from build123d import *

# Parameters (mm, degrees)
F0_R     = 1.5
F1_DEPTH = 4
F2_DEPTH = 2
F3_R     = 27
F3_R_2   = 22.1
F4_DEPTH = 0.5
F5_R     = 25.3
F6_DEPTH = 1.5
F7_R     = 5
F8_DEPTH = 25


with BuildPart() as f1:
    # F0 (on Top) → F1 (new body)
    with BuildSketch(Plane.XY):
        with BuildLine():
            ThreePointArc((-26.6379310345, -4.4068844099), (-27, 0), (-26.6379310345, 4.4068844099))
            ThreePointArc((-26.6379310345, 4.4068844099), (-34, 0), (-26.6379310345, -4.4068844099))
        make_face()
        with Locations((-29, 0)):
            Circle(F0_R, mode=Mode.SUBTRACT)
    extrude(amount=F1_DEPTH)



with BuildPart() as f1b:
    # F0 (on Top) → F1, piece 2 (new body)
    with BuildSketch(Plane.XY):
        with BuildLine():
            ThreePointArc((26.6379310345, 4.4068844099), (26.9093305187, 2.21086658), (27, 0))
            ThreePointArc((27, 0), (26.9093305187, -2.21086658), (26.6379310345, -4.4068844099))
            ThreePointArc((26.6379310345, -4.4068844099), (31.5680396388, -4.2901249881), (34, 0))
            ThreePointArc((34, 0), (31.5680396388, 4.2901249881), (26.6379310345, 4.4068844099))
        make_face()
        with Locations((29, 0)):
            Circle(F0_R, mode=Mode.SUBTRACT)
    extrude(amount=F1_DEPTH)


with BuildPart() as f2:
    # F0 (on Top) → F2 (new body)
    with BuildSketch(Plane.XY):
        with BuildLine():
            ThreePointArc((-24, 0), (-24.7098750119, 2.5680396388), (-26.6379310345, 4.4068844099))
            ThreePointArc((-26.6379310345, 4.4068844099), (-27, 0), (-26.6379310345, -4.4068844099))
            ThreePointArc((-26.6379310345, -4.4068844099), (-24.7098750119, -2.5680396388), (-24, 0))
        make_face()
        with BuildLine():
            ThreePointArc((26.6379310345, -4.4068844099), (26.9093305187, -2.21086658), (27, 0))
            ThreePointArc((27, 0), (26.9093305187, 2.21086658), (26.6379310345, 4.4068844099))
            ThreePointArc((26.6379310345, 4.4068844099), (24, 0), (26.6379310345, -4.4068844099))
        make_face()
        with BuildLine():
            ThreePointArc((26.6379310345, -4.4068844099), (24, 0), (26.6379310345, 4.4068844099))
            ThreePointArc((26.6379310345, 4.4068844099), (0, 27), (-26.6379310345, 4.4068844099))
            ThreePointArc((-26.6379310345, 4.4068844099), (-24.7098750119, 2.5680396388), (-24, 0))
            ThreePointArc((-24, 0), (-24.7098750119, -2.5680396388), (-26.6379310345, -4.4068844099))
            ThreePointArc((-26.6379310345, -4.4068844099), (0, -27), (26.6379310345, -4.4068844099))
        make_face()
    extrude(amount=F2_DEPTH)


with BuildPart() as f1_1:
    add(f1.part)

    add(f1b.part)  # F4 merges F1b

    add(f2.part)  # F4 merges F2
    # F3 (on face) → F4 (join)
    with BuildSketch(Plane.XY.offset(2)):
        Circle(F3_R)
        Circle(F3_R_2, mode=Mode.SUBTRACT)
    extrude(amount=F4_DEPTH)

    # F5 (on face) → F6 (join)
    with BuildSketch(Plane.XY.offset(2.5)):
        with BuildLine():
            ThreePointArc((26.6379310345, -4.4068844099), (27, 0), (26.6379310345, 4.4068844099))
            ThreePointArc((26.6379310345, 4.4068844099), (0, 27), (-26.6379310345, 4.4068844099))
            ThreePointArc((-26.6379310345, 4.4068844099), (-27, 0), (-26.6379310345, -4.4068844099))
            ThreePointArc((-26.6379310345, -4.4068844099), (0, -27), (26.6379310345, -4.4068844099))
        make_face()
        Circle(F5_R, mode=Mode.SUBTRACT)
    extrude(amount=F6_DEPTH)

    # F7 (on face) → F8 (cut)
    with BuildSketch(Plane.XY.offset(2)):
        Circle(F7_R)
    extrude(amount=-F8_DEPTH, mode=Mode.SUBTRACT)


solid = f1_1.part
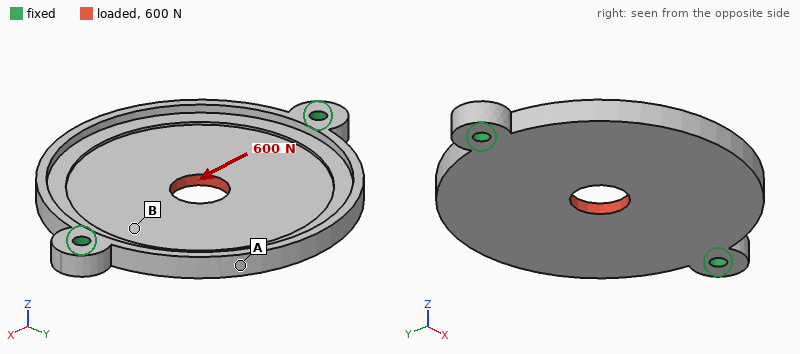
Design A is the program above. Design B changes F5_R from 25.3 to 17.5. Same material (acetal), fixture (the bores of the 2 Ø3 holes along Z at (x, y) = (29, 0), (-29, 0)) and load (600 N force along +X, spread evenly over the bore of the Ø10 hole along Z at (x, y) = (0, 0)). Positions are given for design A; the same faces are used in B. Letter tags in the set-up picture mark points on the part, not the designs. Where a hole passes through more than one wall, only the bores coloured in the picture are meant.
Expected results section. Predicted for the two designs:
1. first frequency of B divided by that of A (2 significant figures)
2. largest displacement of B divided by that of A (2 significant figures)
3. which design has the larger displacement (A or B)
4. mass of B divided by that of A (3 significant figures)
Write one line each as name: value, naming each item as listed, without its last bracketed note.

first frequency of B divided by that of A: 1.1
largest displacement of B divided by that of A: 0.90
which design has the larger displacement: A
mass of B divided by that of A: 1.28
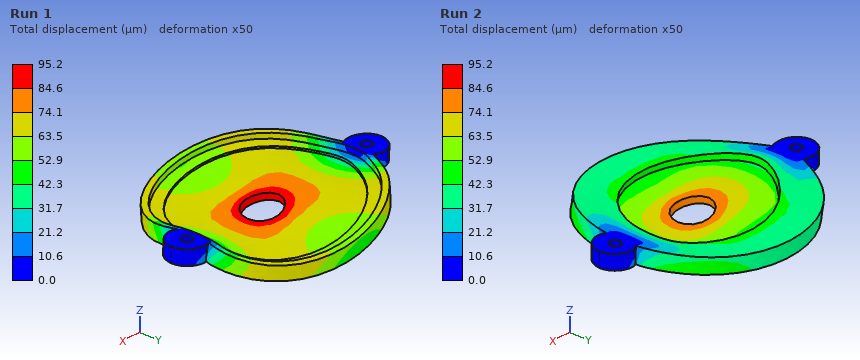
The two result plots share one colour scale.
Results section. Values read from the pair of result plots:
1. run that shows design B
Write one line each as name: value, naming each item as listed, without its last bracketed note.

run that shows design B: Run 2
